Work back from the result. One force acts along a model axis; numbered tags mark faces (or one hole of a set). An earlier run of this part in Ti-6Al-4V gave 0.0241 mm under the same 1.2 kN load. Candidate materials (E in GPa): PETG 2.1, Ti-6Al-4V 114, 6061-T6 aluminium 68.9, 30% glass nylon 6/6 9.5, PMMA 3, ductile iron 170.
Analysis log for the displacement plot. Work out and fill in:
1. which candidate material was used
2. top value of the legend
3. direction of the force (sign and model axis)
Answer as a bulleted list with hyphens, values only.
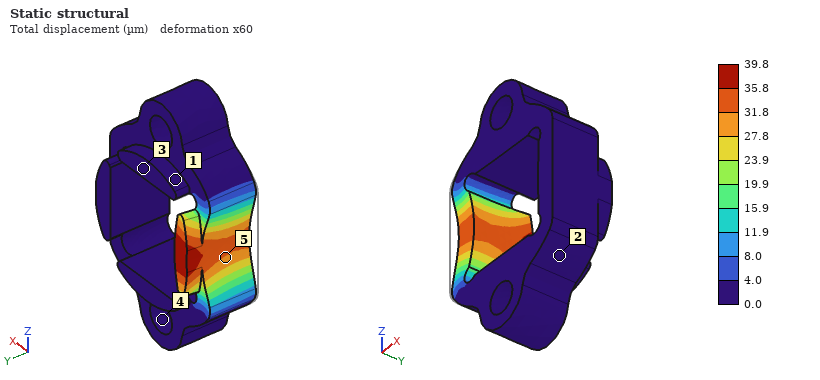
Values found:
- 6061-T6 aluminium
- 39.8 µm
- +X
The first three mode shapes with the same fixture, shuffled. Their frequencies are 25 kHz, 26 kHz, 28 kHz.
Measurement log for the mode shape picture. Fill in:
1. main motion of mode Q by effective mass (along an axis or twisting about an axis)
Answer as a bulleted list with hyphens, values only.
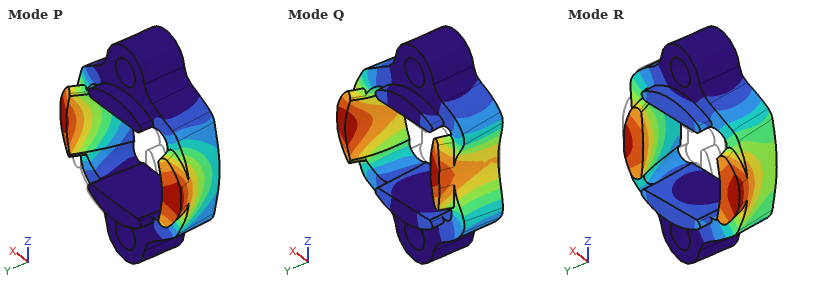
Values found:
- along X
